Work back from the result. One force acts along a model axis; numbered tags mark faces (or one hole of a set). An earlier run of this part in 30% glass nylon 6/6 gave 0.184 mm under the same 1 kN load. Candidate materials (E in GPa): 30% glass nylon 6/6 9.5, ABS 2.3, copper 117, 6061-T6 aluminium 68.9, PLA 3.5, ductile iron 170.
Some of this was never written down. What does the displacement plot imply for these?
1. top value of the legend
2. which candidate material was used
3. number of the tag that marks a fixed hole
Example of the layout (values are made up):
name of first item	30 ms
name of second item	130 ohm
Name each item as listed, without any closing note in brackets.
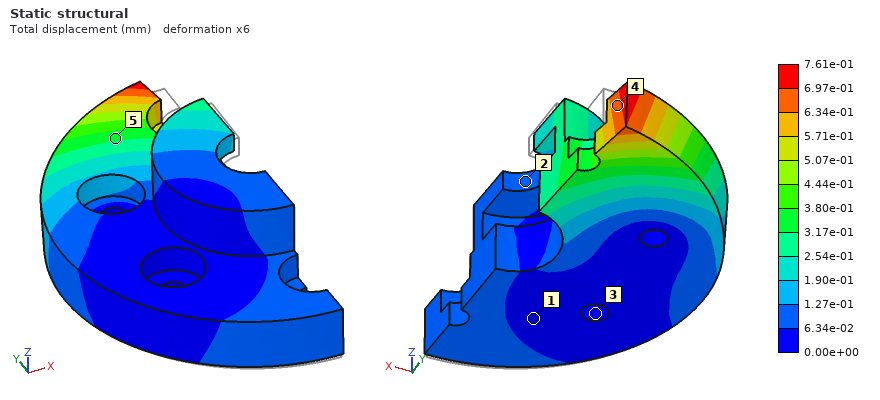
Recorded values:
top value of the legend	7.61e-01 mm
which candidate material was used	ABS
number of the tag that marks a fixed hole	3
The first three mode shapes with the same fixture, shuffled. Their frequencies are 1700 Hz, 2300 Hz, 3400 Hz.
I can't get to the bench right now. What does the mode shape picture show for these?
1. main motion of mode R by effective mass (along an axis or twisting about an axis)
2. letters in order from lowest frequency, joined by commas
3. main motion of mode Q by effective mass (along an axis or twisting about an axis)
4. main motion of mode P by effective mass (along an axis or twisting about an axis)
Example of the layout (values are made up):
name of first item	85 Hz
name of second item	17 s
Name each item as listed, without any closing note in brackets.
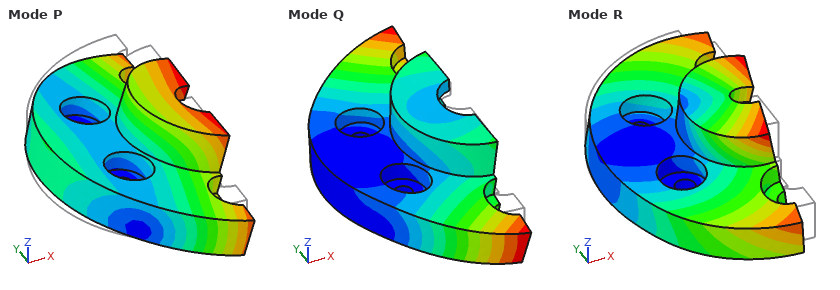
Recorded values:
main motion of mode R by effective mass	along Y
letters in order from lowest frequency, joined by commas	P, Q, R
main motion of mode Q by effective mass	twisting about X
main motion of mode P by effective mass	along Z
